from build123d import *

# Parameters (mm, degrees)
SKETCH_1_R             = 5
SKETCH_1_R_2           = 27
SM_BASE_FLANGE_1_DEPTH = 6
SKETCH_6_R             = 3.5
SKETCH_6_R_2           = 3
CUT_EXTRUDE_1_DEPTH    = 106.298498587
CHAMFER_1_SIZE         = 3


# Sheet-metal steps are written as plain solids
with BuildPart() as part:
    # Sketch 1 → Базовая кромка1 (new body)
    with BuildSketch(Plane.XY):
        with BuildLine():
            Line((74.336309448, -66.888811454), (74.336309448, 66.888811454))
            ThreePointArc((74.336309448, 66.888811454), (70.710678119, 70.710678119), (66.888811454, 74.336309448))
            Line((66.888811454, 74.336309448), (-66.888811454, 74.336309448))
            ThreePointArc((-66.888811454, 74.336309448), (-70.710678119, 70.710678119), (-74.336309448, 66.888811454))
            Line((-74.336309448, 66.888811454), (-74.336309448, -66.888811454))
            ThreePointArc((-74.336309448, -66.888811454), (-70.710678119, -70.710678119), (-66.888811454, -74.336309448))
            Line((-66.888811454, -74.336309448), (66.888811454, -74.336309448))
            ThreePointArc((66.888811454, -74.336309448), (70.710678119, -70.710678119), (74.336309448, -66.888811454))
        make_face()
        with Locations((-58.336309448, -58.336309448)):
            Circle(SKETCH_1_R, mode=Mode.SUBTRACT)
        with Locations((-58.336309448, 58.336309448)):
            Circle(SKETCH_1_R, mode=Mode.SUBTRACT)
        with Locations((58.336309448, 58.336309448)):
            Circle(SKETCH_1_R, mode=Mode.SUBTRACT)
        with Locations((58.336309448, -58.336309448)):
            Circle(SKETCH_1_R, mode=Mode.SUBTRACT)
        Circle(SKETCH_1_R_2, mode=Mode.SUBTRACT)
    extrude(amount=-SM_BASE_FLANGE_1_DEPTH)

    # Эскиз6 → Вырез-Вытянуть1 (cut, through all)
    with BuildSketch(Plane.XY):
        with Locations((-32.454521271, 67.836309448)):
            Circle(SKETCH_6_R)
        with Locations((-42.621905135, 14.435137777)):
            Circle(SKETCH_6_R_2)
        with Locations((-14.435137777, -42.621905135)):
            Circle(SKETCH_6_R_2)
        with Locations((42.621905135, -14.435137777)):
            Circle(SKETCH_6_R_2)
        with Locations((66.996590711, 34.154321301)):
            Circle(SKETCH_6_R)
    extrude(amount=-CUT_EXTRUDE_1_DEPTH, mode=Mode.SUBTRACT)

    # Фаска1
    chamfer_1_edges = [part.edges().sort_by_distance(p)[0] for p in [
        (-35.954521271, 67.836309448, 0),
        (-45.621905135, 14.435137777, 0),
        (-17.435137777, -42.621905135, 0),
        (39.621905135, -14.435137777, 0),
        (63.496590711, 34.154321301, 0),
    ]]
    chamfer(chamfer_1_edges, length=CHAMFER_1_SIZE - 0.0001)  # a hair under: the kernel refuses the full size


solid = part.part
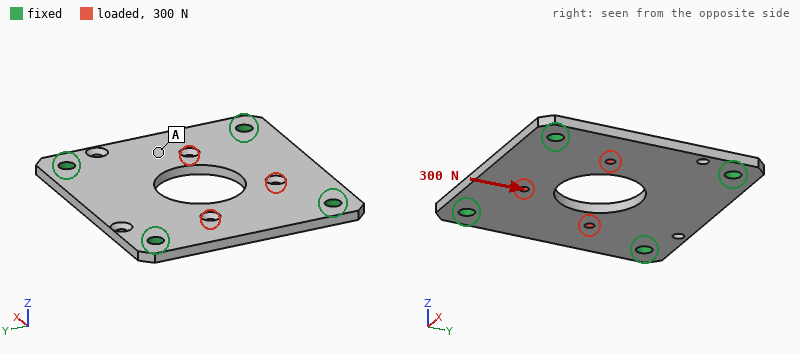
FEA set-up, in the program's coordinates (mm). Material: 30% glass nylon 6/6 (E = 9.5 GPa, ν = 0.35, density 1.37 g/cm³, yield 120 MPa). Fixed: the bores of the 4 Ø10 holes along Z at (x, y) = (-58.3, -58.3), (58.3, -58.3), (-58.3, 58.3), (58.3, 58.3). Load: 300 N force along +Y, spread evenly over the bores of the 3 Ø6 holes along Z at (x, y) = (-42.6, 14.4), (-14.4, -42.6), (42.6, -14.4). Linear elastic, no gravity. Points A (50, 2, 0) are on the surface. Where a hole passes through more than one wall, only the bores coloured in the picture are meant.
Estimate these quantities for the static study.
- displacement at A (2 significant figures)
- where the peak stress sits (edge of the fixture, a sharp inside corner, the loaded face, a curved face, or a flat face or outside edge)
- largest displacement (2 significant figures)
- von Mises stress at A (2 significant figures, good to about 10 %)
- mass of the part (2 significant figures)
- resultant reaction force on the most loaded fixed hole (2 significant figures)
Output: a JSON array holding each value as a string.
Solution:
["3.6 µm", "the loaded face", "5.7 µm", "0.29 MPa", "160 g", "90 N"]
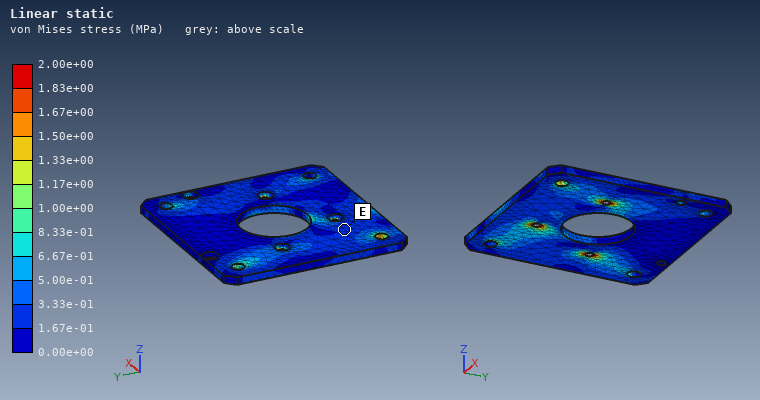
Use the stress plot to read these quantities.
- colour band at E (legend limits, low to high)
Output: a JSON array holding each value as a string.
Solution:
["1.67e-01 to 3.33e-01 MPa"]
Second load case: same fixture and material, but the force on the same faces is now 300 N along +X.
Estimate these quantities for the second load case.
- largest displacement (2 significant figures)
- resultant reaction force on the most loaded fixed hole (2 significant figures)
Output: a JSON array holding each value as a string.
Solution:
["5.3 µm", "99 N"]
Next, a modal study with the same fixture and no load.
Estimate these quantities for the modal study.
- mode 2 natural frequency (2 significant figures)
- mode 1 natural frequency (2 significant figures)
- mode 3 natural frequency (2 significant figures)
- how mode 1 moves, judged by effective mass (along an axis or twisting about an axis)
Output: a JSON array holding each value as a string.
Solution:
["1300 Hz", "940 Hz", "1300 Hz", "along Z"]
